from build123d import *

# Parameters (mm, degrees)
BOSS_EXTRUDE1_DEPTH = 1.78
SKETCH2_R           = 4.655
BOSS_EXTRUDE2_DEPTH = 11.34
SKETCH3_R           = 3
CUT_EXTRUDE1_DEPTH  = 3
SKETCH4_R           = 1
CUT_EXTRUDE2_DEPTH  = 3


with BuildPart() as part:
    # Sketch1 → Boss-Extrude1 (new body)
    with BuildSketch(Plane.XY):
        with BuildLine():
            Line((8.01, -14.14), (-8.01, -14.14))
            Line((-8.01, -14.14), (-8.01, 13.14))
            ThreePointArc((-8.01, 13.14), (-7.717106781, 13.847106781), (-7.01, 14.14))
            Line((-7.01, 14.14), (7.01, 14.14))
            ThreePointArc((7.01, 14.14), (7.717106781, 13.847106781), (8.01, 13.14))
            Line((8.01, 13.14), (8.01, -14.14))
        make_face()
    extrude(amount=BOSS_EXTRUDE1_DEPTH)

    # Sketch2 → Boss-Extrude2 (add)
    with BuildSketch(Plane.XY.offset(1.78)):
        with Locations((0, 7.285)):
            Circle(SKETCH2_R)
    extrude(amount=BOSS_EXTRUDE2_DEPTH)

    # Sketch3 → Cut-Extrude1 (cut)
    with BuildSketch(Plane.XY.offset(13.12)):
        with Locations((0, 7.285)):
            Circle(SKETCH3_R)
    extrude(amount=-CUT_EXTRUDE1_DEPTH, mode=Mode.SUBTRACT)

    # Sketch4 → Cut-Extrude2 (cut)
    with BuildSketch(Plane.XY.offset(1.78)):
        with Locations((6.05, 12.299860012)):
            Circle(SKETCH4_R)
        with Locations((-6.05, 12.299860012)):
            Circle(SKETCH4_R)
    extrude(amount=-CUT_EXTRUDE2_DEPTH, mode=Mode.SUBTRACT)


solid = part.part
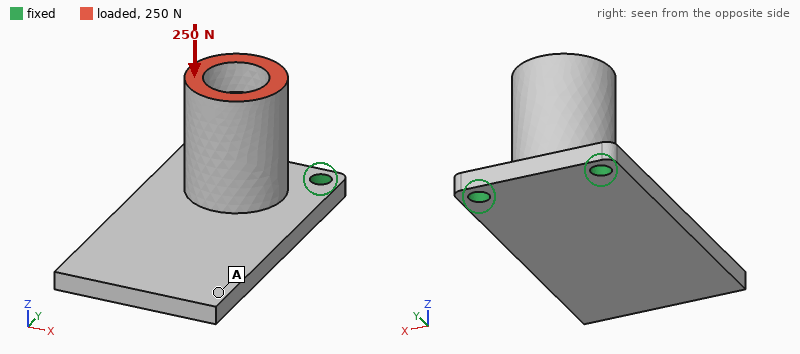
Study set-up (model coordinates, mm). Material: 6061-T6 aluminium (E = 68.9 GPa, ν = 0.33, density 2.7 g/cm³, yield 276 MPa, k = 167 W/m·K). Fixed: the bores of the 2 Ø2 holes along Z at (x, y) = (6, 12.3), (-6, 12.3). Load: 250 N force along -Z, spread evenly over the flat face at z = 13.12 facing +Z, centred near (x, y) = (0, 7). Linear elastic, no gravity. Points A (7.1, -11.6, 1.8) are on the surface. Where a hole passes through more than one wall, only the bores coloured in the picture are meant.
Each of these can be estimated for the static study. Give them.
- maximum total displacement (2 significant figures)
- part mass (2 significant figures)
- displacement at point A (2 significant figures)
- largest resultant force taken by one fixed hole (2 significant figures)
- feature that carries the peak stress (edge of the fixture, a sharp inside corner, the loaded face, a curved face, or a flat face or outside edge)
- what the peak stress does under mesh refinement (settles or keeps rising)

0.14 mm
4.0 g
0.13 mm
130 N
edge of the fixture
keeps rising
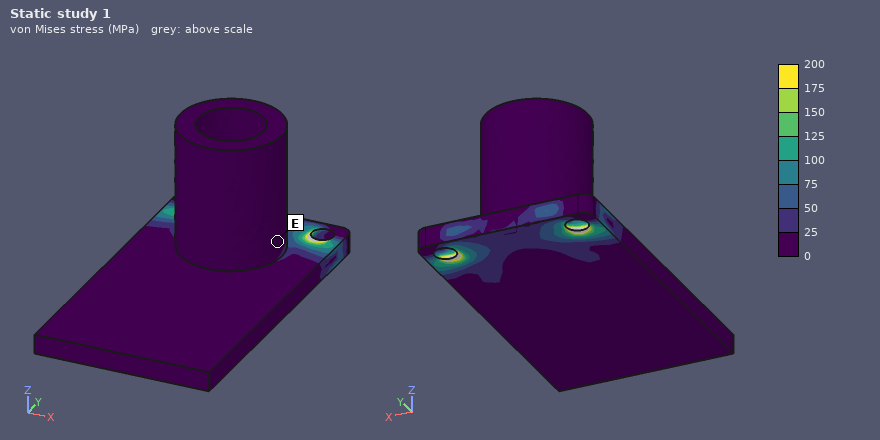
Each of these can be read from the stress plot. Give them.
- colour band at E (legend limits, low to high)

0 to 25 MPa
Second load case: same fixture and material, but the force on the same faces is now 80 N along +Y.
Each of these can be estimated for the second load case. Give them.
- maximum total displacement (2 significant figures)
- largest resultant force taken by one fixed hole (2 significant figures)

0.14 mm
44 N
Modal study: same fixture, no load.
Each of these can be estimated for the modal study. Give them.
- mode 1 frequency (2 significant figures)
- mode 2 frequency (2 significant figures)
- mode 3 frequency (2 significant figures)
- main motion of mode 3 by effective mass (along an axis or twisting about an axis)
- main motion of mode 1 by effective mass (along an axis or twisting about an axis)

2500 Hz
8600 Hz
9200 Hz
twisting about Y
along Z
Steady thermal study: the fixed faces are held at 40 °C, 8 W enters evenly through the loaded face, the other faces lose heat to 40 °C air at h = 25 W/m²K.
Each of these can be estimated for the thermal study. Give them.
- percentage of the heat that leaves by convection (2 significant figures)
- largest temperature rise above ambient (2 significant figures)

3.9 %
18 K
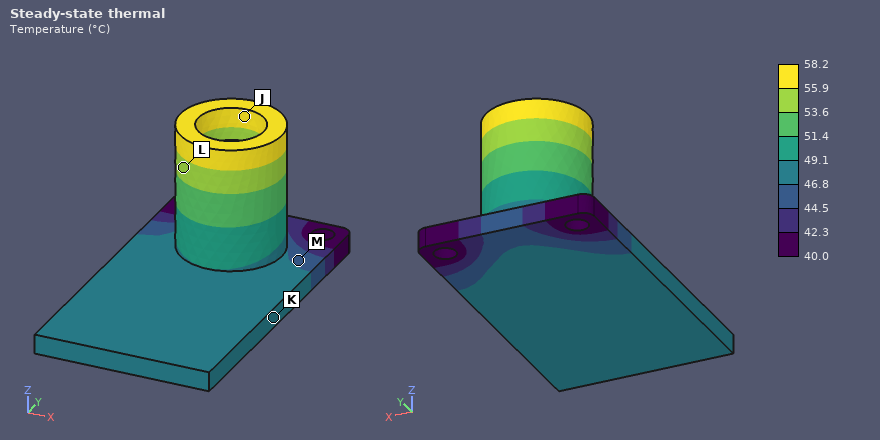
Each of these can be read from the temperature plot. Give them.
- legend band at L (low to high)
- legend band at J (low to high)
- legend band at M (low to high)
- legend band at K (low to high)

53.6 to 55.9 °C
55.9 to 58.2 °C
44.5 to 46.8 °C
46.8 to 49.1 °C
